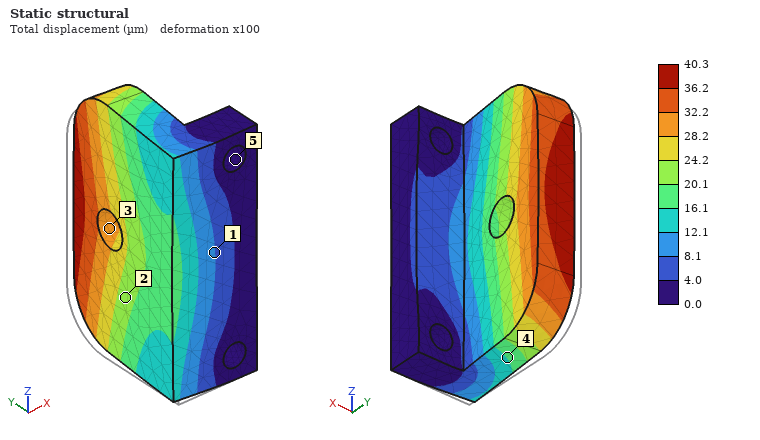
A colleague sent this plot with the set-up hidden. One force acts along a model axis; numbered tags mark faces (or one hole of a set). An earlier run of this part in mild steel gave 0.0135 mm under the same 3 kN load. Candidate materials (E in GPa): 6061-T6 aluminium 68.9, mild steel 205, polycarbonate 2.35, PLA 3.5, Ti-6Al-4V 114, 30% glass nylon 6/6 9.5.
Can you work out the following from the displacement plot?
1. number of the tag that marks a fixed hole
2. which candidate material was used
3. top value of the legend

5
6061-T6 aluminium
40.3 µm
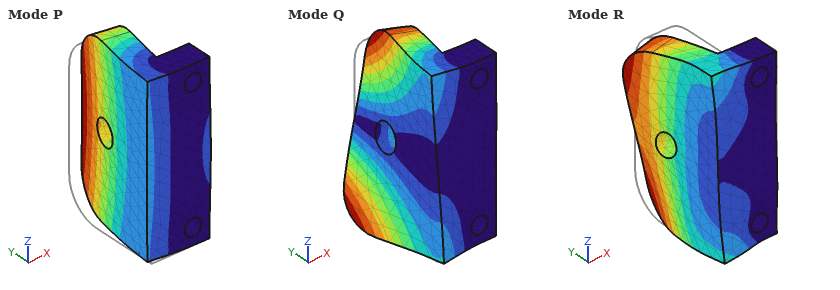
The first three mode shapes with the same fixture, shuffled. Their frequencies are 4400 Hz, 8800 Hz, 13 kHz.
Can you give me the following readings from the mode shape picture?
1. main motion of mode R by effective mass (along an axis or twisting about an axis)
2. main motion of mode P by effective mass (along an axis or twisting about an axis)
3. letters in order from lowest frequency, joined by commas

along Z
along X
P, Q, R
